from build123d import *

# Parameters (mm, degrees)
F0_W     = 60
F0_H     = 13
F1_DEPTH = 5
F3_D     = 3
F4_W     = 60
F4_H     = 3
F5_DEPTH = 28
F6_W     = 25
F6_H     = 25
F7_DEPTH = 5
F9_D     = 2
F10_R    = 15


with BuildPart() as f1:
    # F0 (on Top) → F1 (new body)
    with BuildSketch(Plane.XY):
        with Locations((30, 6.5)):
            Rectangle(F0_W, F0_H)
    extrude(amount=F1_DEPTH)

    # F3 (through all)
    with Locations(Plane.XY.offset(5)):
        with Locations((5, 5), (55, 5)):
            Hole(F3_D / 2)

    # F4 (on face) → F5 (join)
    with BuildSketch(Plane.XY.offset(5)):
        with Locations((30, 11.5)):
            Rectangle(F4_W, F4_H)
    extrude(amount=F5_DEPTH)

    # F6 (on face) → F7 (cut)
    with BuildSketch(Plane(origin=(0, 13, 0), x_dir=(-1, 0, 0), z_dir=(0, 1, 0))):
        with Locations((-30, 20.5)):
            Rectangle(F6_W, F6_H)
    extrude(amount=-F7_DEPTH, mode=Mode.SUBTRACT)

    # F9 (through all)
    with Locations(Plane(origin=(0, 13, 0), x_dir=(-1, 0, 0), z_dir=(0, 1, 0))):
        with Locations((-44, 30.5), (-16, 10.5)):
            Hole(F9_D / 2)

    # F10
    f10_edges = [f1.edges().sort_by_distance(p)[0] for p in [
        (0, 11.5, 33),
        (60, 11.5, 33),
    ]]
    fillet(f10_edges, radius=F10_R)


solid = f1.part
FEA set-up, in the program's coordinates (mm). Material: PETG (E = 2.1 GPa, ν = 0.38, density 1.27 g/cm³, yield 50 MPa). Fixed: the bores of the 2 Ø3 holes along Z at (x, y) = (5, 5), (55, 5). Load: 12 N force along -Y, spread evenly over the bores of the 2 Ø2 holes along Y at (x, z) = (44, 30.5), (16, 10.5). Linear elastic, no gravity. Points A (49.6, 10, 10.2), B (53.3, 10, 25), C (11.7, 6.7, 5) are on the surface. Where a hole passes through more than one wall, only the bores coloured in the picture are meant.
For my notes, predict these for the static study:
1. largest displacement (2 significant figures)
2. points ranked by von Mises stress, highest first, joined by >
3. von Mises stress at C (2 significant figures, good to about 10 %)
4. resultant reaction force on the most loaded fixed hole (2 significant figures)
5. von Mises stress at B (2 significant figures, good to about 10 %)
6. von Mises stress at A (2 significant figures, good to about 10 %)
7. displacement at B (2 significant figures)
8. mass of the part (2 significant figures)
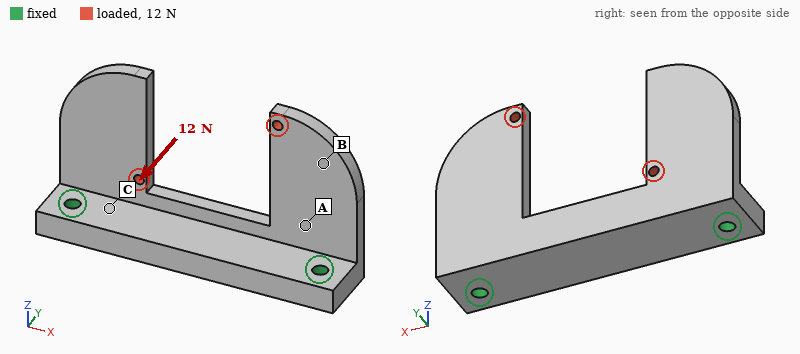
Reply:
0.68 mm
A > B > C
1.0 MPa
6.9 N
2.0 MPa
4.4 MPa
0.35 mm
8.5 g
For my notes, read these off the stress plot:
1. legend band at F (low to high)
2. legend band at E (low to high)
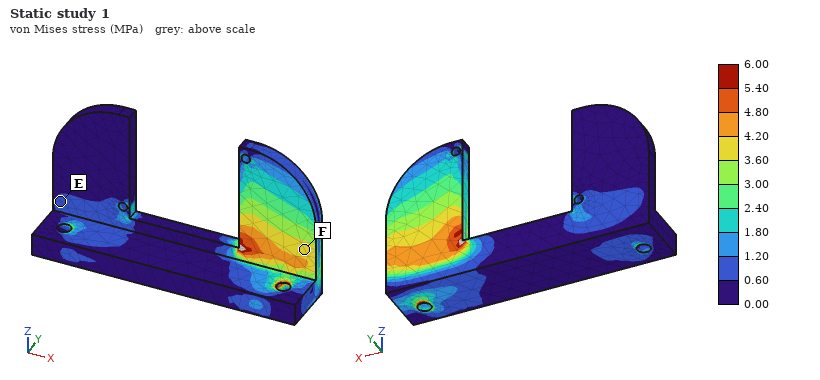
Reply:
3.60 to 4.20 MPa
0.60 to 1.20 MPa
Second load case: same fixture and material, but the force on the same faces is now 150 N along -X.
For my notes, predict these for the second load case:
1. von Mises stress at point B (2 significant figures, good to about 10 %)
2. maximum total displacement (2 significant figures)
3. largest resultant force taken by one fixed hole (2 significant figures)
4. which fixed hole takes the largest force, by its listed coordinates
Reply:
3.8 MPa
0.75 mm
100 N
(5, 5)
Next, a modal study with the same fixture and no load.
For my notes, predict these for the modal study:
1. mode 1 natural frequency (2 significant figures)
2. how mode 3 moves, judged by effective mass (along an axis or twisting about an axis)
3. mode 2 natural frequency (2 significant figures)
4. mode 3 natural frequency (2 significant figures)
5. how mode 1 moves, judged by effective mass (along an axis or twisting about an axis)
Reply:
770 Hz
along Z
810 Hz
1600 Hz
along Y
